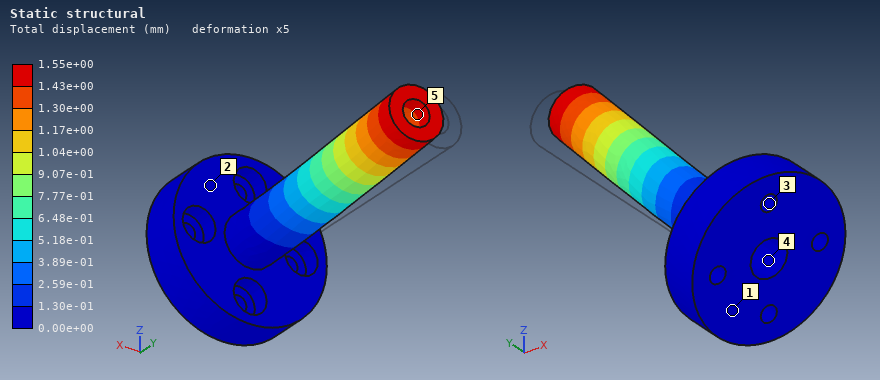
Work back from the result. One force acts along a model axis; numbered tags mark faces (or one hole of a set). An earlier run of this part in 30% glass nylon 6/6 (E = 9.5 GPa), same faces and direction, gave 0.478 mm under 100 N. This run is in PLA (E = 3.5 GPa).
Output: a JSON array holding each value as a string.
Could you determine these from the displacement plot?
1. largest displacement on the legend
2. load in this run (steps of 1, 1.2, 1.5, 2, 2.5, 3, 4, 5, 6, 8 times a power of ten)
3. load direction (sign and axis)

["1.55e+00 mm", "120 N", "+X"]
